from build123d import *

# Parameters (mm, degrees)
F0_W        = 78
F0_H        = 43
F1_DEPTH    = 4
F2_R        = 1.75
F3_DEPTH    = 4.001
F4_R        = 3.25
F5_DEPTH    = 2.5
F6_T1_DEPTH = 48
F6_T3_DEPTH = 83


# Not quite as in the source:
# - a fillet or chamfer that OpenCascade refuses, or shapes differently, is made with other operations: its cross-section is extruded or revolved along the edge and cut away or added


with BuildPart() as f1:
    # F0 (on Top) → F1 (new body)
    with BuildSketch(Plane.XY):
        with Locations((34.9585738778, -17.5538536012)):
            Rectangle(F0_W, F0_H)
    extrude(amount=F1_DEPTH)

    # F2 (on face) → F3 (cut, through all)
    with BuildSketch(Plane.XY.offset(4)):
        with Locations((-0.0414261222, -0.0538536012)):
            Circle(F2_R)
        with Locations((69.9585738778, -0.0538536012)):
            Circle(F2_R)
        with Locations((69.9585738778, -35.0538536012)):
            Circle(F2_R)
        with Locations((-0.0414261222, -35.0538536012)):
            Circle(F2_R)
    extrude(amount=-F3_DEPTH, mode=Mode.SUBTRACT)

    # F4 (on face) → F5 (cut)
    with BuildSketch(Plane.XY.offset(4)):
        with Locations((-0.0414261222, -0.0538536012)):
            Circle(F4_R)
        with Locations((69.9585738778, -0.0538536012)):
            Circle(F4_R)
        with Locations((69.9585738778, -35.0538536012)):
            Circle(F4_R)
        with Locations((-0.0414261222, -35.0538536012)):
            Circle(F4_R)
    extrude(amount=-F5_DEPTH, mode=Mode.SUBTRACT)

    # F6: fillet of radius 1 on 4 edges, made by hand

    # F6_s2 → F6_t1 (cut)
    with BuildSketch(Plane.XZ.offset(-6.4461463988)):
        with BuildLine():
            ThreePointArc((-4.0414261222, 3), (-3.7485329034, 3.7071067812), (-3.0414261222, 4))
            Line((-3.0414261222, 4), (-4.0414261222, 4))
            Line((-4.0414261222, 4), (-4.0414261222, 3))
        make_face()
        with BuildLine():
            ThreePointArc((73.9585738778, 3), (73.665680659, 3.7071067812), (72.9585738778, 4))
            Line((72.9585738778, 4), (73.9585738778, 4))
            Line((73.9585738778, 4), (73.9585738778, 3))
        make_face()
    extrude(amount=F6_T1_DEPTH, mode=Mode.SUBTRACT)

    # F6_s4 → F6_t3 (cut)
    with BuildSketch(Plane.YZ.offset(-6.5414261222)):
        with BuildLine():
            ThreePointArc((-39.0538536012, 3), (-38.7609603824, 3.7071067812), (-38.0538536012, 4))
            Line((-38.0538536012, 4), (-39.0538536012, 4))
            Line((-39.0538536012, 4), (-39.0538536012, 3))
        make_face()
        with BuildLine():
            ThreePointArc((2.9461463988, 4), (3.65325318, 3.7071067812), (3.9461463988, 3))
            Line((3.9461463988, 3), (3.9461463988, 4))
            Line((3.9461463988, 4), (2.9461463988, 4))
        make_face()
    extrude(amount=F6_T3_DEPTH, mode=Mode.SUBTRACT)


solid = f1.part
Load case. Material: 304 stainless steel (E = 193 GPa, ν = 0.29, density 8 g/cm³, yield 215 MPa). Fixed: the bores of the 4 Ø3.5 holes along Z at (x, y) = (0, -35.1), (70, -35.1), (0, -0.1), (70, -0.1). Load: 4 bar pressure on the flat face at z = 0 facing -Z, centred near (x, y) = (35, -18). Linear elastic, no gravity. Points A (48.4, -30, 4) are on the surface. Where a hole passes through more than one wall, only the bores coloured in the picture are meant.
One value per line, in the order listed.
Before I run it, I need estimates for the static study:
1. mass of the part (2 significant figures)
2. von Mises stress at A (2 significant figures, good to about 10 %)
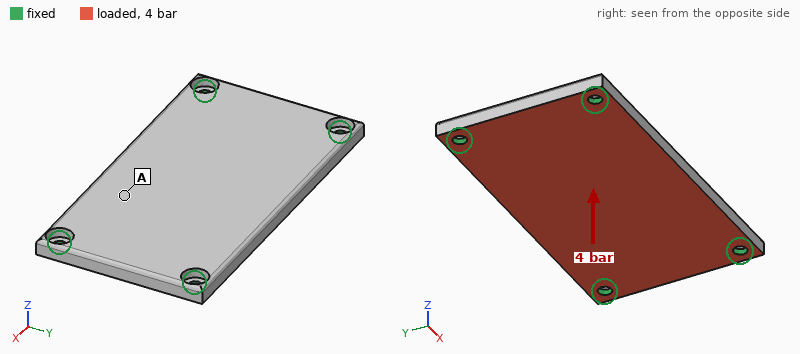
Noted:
100 g
39 MPa
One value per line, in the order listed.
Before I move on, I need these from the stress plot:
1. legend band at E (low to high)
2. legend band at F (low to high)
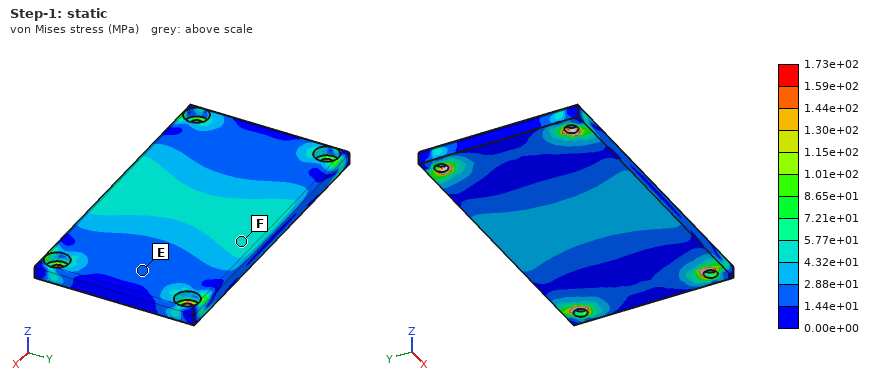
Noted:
1.44e+01 to 2.88e+01 MPa
4.32e+01 to 5.77e+01 MPa
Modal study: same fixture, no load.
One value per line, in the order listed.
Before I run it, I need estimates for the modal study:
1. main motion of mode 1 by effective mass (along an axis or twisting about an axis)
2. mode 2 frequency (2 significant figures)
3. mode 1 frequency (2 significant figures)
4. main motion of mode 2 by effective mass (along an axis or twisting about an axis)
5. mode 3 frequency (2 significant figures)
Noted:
along Z
5200 Hz
2900 Hz
twisting about X
7900 Hz
